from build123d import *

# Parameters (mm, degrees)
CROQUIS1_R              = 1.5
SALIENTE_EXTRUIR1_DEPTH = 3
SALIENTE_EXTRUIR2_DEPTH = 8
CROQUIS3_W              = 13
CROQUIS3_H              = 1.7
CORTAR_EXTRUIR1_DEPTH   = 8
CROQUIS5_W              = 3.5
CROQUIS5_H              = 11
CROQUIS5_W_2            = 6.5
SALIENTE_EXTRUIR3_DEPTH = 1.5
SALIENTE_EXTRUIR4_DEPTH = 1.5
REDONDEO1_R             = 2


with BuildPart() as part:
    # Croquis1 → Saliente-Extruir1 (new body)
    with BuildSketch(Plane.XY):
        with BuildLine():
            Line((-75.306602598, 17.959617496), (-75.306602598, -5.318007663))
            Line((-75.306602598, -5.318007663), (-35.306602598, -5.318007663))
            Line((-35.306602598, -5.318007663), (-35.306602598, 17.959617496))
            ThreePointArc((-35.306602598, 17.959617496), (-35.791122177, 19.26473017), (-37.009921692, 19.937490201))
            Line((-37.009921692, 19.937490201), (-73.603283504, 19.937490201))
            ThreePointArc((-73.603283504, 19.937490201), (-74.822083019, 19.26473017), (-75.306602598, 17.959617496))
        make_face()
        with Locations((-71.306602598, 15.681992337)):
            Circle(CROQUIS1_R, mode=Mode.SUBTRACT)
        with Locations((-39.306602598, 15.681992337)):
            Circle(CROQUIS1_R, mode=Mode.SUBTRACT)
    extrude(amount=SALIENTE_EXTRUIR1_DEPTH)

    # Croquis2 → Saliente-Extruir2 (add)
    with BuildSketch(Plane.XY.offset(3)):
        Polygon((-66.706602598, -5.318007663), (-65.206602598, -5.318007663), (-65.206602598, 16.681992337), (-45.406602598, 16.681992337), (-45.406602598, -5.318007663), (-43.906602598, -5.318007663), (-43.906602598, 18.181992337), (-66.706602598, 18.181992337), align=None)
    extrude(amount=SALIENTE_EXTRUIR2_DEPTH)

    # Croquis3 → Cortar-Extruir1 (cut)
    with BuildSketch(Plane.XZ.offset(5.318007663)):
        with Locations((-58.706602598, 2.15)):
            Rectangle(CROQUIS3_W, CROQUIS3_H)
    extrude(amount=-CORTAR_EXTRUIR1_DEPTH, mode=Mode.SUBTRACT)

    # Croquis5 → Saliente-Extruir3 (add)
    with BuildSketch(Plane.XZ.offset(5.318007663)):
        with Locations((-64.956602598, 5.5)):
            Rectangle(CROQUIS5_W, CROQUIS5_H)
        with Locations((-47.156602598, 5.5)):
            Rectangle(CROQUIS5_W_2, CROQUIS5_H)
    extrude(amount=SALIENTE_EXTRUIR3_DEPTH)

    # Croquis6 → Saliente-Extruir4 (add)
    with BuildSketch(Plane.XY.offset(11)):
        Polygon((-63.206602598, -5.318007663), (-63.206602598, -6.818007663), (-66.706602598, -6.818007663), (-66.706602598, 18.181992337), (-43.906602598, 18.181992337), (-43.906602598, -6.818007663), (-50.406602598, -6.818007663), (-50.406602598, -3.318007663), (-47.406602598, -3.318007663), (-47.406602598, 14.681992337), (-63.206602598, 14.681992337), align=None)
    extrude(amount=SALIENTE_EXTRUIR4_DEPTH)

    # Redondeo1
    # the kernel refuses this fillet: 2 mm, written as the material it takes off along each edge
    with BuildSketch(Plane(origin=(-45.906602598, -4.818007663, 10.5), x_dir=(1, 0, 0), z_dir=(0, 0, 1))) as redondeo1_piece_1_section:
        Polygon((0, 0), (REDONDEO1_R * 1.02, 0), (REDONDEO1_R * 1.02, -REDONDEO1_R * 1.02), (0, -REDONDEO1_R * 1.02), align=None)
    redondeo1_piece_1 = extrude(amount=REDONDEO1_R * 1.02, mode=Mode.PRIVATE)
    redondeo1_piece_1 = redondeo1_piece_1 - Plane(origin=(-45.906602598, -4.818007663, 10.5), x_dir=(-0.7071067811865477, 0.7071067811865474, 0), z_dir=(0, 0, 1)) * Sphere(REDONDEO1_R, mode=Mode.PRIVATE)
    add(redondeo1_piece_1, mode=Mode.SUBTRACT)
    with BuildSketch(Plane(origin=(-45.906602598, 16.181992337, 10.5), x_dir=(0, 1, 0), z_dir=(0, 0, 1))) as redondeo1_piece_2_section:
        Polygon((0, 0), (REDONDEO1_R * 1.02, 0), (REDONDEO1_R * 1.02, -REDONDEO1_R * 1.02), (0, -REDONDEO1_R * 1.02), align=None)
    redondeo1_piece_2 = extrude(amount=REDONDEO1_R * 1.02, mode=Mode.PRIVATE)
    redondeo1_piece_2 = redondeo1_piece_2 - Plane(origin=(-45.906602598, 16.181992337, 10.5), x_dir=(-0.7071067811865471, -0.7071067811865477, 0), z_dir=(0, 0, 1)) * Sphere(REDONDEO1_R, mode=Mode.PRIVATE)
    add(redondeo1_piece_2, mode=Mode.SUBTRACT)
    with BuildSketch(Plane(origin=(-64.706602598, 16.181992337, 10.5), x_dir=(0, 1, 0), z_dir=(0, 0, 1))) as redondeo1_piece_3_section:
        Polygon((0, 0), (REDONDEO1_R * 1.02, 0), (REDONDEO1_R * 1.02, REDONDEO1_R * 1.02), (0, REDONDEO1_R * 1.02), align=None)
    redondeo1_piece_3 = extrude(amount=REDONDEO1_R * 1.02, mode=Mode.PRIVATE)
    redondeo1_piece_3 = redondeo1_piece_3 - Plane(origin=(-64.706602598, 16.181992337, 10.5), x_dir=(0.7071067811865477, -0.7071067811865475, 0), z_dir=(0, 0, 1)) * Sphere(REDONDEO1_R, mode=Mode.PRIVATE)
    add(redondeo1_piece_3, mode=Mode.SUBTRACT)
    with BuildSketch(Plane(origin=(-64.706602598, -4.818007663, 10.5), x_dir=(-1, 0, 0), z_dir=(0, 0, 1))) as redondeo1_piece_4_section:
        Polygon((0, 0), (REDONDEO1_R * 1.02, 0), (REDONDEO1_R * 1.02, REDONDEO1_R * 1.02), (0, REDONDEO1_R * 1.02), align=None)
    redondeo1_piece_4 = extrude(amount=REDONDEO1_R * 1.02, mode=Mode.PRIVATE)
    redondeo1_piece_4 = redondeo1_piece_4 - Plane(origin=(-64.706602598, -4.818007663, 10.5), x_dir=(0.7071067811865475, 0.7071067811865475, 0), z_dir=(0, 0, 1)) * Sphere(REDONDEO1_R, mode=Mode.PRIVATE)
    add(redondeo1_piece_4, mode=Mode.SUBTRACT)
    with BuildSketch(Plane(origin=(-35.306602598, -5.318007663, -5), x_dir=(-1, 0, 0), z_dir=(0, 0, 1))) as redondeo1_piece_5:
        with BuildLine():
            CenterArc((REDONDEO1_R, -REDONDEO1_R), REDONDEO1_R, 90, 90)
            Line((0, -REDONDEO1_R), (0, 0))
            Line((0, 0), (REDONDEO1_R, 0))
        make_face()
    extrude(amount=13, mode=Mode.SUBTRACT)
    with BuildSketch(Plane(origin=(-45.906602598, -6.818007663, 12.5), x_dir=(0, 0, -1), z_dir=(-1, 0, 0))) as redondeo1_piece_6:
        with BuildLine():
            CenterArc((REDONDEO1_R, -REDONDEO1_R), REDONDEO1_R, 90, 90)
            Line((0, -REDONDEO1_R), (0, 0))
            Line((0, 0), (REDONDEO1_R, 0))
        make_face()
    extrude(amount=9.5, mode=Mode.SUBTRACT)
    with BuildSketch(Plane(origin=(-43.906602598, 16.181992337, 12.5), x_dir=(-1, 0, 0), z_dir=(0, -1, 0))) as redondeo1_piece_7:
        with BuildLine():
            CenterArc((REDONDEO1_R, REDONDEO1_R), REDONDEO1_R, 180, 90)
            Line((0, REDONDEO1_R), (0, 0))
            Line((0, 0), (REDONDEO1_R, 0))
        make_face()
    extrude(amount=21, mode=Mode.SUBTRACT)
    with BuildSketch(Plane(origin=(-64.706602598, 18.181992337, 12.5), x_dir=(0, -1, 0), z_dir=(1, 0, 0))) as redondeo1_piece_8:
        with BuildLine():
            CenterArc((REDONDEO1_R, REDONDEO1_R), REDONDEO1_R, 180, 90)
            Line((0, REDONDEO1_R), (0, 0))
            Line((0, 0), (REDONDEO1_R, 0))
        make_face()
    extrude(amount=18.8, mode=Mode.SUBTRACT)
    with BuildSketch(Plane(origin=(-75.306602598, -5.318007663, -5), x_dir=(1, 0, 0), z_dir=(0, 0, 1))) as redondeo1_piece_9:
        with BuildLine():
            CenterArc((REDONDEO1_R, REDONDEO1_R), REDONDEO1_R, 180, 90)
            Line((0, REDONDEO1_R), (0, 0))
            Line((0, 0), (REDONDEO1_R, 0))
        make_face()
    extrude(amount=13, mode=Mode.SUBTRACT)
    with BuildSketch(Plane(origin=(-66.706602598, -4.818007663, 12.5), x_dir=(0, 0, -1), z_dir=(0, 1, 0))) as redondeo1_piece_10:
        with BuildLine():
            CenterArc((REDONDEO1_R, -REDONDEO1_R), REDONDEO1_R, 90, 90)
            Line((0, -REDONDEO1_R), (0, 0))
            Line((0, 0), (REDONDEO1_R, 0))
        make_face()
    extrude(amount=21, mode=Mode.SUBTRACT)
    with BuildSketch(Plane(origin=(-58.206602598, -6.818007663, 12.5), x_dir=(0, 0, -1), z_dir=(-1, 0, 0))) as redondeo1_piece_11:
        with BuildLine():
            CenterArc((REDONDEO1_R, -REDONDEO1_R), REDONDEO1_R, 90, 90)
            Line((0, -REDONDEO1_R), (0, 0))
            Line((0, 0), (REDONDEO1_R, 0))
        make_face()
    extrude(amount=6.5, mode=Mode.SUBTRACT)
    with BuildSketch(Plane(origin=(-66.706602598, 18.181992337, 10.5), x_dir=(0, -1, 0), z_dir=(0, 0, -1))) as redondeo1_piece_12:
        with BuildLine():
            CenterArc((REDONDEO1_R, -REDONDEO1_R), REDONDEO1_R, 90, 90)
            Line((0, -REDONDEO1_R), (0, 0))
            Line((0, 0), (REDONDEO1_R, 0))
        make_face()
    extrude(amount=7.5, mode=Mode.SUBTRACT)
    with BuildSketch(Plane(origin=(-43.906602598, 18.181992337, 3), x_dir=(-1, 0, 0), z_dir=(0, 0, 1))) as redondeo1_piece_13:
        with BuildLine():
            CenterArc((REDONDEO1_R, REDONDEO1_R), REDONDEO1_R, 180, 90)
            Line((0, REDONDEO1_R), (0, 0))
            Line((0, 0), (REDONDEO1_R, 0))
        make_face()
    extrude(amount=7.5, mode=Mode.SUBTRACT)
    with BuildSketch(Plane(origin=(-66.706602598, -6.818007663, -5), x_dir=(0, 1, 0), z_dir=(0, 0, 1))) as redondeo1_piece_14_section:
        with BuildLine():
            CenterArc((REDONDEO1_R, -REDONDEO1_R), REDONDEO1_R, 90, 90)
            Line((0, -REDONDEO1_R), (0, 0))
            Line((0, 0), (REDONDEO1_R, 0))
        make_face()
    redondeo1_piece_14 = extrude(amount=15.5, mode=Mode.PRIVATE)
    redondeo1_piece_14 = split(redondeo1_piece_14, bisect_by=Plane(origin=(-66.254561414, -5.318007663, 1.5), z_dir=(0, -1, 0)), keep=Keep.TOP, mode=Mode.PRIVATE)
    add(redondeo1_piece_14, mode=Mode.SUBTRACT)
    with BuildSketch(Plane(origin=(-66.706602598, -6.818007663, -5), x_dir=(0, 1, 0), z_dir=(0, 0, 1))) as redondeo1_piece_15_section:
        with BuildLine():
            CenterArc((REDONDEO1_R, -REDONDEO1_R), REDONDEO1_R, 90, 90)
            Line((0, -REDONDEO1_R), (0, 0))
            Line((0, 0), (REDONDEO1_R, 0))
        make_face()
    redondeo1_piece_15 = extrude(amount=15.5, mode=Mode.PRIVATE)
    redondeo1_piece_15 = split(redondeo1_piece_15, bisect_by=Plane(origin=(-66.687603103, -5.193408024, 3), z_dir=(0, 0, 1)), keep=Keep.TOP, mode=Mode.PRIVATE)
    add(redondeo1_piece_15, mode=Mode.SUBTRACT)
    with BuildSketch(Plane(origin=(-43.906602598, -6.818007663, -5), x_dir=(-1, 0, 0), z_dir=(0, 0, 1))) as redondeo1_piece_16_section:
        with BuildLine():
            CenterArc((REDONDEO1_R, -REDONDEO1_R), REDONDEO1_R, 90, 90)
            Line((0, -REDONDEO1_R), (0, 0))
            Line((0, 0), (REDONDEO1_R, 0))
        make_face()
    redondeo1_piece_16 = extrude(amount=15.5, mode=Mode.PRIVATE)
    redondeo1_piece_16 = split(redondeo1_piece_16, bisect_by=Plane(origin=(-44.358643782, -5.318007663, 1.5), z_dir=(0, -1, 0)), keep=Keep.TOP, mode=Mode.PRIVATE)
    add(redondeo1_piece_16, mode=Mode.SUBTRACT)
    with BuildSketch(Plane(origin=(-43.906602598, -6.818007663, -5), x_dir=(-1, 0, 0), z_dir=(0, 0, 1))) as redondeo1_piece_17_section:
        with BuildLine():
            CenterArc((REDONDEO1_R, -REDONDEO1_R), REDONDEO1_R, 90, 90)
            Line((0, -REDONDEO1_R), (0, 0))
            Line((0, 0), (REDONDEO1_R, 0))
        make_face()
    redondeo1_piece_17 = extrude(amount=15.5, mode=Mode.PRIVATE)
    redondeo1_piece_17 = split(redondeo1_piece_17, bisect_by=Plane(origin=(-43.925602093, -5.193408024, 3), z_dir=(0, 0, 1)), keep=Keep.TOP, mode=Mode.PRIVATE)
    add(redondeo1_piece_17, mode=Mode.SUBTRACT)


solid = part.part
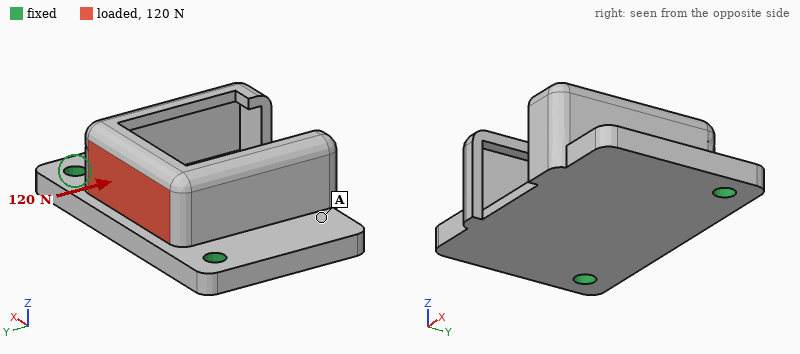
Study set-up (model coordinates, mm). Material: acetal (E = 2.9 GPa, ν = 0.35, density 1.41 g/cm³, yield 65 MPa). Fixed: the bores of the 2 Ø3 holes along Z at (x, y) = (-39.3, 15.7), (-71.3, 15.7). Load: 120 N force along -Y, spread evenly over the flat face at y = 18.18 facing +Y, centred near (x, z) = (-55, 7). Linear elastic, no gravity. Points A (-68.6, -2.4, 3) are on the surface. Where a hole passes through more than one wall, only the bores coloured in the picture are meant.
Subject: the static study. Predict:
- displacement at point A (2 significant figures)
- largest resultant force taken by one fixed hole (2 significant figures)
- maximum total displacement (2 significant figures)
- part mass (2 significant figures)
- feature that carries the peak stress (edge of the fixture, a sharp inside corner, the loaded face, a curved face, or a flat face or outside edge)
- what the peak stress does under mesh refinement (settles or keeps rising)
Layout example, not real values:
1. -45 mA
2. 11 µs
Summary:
1. 0.23 mm
2. 63 N
3. 0.33 mm
4. 5.7 g
5. edge of the fixture
6. keeps rising
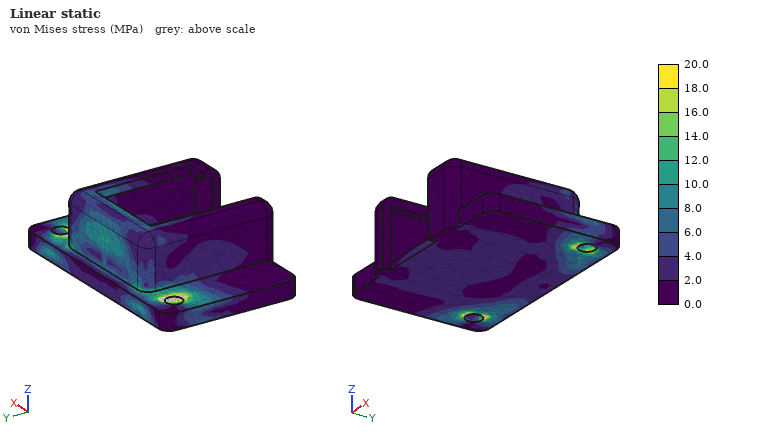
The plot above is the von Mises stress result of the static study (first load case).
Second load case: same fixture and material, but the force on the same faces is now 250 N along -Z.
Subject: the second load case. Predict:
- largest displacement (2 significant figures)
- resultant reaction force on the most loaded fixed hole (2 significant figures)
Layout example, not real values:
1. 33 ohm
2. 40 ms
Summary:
1. 0.33 mm
2. 140 N
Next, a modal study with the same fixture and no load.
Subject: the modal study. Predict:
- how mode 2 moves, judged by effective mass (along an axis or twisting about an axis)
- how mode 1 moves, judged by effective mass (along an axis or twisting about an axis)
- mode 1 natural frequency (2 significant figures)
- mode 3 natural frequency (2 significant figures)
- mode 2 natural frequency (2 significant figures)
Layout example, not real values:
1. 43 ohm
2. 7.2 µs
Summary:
1. twisting about Y
2. along Z
3. 1200 Hz
4. 2800 Hz
5. 2200 Hz
